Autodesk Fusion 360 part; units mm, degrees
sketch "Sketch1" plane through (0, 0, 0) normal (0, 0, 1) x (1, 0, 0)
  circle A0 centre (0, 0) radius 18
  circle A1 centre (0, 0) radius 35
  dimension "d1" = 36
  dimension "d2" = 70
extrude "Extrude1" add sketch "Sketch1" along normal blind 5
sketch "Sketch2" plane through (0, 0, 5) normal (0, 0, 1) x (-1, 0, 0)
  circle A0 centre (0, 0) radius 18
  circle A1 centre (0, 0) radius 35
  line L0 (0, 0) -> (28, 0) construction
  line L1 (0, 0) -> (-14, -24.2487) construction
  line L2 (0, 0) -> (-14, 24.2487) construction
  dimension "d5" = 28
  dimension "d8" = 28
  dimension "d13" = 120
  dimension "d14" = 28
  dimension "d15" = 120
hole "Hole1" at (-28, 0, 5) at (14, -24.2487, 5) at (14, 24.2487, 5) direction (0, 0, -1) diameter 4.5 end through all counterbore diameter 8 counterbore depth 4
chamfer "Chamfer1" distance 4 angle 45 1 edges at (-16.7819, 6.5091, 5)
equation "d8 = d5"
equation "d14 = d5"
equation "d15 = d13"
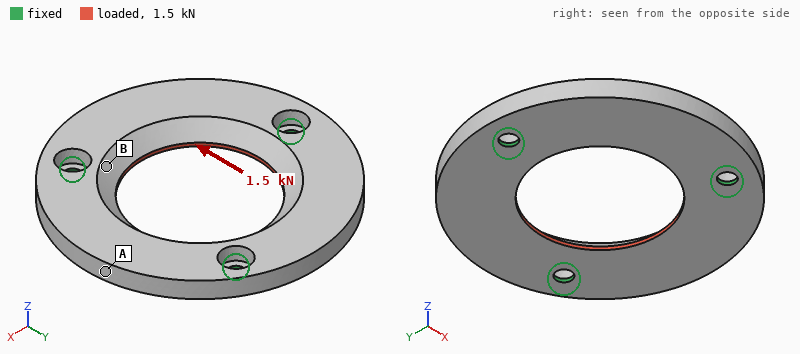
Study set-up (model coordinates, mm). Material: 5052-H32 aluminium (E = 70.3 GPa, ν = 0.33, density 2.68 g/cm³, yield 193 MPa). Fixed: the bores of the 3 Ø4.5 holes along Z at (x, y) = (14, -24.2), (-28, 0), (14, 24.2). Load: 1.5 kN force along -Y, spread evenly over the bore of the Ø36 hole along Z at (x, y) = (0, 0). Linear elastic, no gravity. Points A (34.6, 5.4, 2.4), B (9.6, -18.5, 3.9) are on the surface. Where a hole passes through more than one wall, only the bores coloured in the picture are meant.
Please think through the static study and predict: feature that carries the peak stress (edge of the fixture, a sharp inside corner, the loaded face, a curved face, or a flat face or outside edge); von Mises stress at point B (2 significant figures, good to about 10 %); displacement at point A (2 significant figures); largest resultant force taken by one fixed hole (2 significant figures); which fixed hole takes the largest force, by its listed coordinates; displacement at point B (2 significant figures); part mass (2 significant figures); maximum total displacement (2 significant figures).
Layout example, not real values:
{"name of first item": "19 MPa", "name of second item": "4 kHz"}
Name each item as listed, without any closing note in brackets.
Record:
{"feature that carries the peak stress": "edge of the fixture", "von Mises stress at point B": "11 MPa", "displacement at point A": "2.9 µm", "largest resultant force taken by one fixed hole": "600 N", "which fixed hole takes the largest force, by its listed coordinates": "(-28, 0)", "displacement at point B": "3.0 µm", "part mass": "34 g", "maximum total displacement": "8.6 µm"}
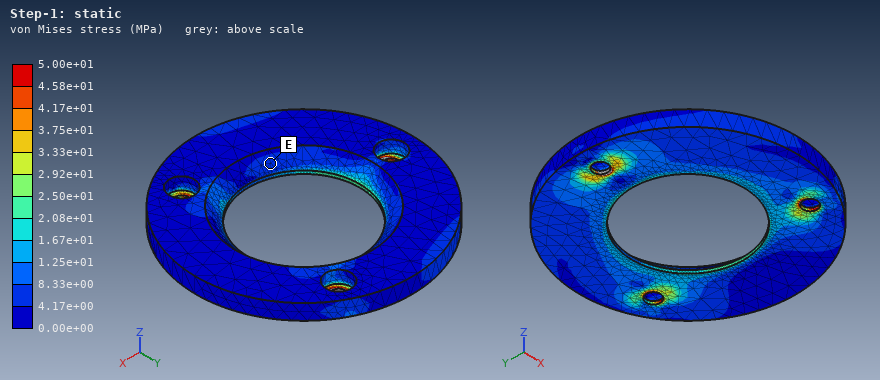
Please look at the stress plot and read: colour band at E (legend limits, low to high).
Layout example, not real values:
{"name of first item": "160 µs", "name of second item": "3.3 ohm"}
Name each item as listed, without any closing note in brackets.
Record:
{"colour band at E": "4.17e+00 to 8.33e+00 MPa"}
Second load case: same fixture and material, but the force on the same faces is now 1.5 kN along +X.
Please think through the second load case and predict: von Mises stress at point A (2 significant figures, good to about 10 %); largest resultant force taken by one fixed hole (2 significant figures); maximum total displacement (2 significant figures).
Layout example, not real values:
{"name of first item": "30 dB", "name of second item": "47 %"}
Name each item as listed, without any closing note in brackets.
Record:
{"von Mises stress at point A": "6.0 MPa", "largest resultant force taken by one fixed hole": "560 N", "maximum total displacement": "9.4 µm"}
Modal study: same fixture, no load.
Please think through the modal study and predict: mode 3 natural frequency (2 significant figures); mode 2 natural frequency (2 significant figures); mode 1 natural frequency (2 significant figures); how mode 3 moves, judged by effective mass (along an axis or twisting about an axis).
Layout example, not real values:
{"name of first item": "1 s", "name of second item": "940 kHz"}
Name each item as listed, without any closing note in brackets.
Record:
{"mode 3 natural frequency": "5600 Hz", "mode 2 natural frequency": "3400 Hz", "mode 1 natural frequency": "3400 Hz", "how mode 3 moves, judged by effective mass": "along Z"}
